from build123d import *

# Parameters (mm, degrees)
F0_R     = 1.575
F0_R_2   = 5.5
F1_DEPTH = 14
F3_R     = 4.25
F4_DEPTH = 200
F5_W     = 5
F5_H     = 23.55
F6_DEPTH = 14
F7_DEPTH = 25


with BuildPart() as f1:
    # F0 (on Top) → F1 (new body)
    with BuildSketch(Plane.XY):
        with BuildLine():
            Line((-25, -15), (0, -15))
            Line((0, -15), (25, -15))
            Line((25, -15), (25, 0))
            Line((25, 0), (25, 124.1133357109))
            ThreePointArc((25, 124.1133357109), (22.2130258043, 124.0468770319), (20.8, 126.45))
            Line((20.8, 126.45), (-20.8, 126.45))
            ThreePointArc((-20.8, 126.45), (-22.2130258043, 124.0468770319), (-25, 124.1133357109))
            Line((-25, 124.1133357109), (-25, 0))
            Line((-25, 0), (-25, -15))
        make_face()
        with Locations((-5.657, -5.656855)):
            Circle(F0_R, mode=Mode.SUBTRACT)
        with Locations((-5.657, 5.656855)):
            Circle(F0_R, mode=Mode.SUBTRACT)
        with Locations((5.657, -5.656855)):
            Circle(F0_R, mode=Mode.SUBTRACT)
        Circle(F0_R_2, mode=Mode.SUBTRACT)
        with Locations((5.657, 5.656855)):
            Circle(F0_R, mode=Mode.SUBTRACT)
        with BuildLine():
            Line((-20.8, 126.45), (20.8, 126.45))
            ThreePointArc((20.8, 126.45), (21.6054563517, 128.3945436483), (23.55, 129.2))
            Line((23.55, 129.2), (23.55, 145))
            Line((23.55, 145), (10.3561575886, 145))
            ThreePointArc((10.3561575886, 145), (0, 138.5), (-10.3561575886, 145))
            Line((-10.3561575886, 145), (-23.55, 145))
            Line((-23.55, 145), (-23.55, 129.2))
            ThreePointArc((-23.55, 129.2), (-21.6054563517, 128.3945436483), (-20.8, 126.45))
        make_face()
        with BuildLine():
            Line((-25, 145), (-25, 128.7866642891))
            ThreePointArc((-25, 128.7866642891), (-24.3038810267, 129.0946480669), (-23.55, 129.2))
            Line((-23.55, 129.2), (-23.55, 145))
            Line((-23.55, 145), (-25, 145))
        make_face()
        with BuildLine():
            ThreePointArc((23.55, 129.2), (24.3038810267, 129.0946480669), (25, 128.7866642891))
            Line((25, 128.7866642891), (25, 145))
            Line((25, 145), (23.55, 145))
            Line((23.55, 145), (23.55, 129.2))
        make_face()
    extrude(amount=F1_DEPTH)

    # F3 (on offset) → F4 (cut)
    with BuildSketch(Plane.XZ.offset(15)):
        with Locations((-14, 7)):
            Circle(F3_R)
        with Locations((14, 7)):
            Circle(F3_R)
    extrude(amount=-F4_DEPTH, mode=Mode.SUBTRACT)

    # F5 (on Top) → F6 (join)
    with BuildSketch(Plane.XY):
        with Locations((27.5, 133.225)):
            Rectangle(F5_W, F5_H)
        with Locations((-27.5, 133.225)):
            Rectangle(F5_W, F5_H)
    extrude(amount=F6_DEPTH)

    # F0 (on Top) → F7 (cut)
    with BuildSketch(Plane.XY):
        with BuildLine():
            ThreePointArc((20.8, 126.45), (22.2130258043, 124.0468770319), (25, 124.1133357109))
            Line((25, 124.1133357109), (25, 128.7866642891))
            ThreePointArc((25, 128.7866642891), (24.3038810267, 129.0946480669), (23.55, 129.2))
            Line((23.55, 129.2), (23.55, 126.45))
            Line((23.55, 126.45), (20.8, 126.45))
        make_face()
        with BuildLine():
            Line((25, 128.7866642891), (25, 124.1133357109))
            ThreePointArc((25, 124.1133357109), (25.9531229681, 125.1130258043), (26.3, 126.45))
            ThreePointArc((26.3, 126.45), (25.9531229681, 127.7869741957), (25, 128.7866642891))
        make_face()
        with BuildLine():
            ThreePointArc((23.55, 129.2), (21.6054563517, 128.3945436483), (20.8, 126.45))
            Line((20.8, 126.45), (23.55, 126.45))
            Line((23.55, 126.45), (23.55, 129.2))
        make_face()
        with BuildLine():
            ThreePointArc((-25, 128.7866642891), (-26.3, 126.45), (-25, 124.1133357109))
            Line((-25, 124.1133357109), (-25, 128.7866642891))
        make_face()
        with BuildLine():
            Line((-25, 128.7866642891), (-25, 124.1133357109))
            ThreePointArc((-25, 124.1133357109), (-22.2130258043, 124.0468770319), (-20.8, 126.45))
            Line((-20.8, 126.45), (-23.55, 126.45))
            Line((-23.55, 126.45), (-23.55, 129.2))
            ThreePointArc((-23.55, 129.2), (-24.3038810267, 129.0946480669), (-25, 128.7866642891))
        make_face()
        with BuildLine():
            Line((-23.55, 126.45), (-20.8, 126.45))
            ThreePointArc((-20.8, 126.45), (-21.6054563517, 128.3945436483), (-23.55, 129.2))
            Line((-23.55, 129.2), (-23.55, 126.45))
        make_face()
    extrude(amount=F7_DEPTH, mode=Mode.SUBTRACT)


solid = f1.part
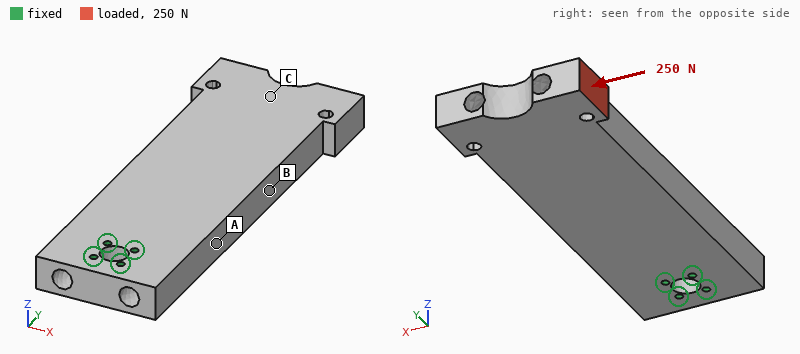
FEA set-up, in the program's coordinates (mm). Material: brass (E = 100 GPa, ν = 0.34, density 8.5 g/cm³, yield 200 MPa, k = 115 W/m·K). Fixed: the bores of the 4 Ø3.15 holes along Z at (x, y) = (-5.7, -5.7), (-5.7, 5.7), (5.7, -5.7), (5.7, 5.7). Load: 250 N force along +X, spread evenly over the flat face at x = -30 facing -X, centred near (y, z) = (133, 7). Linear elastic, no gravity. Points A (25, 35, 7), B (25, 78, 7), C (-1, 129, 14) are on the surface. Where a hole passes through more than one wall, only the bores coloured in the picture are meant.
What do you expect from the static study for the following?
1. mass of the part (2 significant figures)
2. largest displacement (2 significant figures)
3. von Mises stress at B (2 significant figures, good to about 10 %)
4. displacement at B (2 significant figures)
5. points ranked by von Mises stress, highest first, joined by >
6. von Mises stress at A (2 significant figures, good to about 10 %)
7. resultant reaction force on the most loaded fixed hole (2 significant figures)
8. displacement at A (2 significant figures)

790 g
33 µm
2.8 MPa
15 µm
A > B > C
5.1 MPa
1.2 kN
6.1 µm
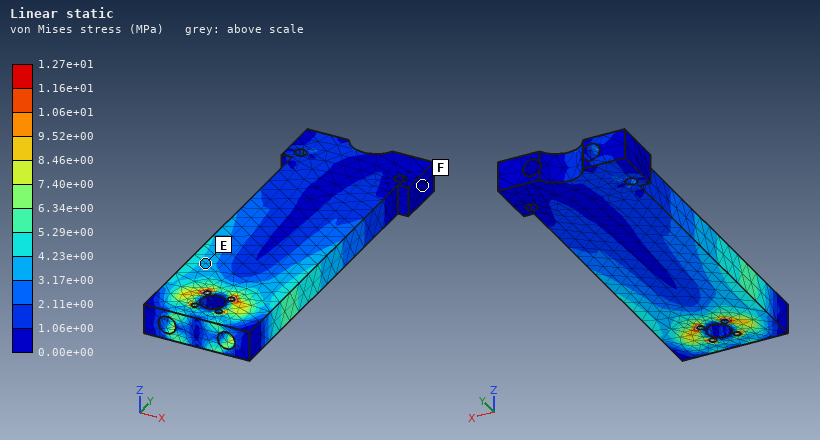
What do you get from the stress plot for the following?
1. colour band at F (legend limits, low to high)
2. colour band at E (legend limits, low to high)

0.00e+00 to 1.06e+00 MPa
3.17e+00 to 4.23e+00 MPa
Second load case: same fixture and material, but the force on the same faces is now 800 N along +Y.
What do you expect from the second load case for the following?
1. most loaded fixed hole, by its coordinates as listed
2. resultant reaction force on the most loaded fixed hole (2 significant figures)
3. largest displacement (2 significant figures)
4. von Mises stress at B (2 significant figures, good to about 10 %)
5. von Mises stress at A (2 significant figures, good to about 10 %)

(-5.7, 5.7)
1.2 kN
34 µm
3.5 MPa
3.8 MPa
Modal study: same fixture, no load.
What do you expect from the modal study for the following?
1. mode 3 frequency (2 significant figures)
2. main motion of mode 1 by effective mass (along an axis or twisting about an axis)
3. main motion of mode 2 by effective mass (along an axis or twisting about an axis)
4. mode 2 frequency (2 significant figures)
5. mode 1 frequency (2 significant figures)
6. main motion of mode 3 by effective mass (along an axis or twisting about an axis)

1700 Hz
along Z
along X
910 Hz
390 Hz
twisting about Y
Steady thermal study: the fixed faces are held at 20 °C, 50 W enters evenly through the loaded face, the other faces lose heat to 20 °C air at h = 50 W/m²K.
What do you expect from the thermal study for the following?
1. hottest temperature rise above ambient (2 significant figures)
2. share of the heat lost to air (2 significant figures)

80 K
66 %
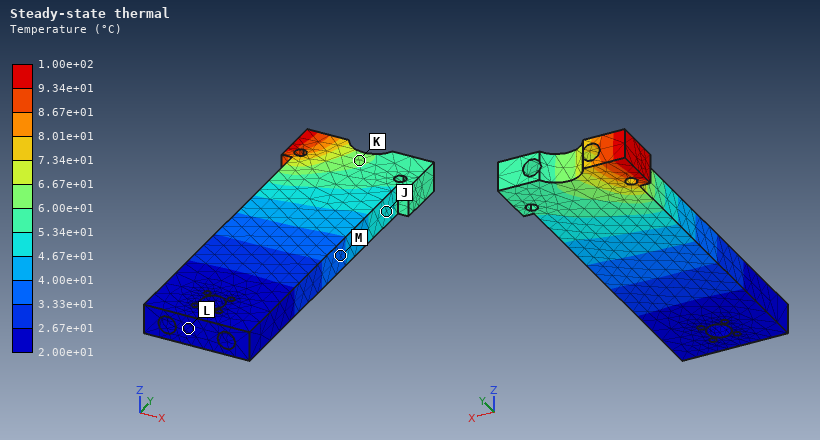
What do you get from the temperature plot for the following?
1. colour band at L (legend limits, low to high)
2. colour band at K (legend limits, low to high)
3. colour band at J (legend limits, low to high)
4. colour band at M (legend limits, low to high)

2.00e+01 to 2.67e+01 °C
6.00e+01 to 6.67e+01 °C
4.67e+01 to 5.34e+01 °C
3.33e+01 to 4.00e+01 °C
